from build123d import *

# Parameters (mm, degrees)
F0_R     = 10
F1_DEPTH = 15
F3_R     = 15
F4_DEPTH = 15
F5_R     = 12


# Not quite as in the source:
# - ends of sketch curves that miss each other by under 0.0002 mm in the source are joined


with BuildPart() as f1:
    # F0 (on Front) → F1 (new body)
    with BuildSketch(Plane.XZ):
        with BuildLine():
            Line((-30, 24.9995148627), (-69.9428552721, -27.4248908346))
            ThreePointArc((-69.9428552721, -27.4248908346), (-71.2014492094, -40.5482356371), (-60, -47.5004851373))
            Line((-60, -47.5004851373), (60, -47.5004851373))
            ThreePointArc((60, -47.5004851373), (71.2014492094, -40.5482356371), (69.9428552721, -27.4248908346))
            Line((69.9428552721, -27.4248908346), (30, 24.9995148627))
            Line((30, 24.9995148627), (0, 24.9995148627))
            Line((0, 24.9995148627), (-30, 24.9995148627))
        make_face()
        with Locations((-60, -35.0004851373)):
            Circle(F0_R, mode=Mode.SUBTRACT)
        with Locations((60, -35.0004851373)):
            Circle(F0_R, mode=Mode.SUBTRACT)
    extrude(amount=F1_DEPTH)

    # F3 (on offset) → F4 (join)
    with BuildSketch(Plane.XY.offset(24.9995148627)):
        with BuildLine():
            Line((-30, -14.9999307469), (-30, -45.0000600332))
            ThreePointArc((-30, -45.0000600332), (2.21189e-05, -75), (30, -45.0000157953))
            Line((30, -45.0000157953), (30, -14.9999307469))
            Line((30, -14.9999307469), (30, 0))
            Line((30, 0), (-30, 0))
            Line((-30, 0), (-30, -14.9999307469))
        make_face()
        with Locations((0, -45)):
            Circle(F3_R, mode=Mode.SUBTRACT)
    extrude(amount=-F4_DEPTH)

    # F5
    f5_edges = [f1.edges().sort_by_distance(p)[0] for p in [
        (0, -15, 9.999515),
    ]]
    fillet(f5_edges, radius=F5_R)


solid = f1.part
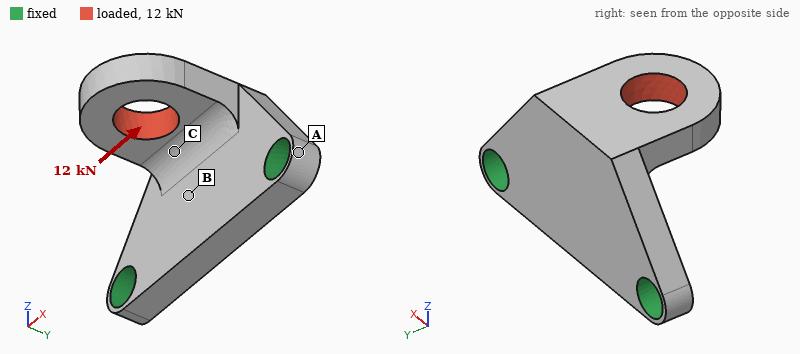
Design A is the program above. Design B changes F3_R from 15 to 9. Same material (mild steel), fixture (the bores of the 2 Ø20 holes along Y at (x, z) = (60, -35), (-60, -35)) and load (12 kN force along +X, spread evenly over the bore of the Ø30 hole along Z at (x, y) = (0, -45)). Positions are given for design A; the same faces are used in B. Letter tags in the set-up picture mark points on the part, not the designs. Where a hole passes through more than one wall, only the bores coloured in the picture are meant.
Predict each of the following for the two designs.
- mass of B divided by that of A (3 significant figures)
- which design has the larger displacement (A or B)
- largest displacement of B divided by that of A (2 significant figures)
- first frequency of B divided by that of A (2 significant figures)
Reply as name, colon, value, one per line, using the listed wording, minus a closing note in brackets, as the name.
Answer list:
mass of B divided by that of A: 1.04
which design has the larger displacement: A
largest displacement of B divided by that of A: 0.90
first frequency of B divided by that of A: 0.95
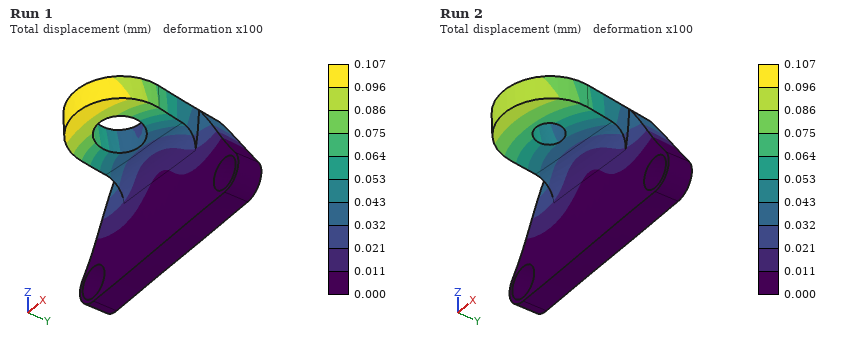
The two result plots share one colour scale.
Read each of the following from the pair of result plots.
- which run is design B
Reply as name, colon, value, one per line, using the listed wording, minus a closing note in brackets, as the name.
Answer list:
which run is design B: Run 2
